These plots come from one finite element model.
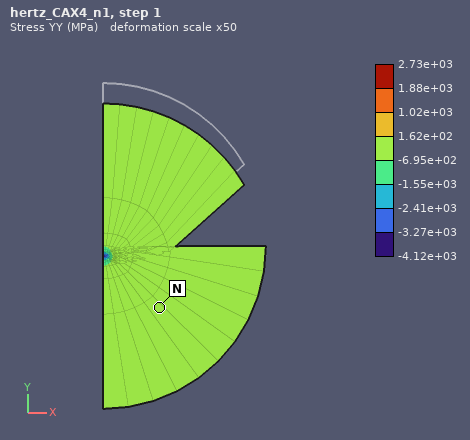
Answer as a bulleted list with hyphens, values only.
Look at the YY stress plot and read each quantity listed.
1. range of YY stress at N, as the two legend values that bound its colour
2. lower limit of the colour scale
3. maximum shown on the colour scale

- -6.95e+02 to 1.62e+02 MPa
- -4.12e+03 MPa
- 2.73e+03 MPa
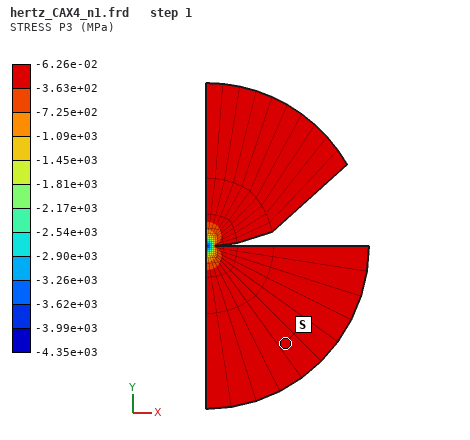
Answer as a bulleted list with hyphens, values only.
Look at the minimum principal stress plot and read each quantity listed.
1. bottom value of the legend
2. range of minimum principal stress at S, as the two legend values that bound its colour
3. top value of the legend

- -4.35e+03 MPa
- -3.63e+02 to -6.26e-02 MPa
- -6.26e-02 MPa
